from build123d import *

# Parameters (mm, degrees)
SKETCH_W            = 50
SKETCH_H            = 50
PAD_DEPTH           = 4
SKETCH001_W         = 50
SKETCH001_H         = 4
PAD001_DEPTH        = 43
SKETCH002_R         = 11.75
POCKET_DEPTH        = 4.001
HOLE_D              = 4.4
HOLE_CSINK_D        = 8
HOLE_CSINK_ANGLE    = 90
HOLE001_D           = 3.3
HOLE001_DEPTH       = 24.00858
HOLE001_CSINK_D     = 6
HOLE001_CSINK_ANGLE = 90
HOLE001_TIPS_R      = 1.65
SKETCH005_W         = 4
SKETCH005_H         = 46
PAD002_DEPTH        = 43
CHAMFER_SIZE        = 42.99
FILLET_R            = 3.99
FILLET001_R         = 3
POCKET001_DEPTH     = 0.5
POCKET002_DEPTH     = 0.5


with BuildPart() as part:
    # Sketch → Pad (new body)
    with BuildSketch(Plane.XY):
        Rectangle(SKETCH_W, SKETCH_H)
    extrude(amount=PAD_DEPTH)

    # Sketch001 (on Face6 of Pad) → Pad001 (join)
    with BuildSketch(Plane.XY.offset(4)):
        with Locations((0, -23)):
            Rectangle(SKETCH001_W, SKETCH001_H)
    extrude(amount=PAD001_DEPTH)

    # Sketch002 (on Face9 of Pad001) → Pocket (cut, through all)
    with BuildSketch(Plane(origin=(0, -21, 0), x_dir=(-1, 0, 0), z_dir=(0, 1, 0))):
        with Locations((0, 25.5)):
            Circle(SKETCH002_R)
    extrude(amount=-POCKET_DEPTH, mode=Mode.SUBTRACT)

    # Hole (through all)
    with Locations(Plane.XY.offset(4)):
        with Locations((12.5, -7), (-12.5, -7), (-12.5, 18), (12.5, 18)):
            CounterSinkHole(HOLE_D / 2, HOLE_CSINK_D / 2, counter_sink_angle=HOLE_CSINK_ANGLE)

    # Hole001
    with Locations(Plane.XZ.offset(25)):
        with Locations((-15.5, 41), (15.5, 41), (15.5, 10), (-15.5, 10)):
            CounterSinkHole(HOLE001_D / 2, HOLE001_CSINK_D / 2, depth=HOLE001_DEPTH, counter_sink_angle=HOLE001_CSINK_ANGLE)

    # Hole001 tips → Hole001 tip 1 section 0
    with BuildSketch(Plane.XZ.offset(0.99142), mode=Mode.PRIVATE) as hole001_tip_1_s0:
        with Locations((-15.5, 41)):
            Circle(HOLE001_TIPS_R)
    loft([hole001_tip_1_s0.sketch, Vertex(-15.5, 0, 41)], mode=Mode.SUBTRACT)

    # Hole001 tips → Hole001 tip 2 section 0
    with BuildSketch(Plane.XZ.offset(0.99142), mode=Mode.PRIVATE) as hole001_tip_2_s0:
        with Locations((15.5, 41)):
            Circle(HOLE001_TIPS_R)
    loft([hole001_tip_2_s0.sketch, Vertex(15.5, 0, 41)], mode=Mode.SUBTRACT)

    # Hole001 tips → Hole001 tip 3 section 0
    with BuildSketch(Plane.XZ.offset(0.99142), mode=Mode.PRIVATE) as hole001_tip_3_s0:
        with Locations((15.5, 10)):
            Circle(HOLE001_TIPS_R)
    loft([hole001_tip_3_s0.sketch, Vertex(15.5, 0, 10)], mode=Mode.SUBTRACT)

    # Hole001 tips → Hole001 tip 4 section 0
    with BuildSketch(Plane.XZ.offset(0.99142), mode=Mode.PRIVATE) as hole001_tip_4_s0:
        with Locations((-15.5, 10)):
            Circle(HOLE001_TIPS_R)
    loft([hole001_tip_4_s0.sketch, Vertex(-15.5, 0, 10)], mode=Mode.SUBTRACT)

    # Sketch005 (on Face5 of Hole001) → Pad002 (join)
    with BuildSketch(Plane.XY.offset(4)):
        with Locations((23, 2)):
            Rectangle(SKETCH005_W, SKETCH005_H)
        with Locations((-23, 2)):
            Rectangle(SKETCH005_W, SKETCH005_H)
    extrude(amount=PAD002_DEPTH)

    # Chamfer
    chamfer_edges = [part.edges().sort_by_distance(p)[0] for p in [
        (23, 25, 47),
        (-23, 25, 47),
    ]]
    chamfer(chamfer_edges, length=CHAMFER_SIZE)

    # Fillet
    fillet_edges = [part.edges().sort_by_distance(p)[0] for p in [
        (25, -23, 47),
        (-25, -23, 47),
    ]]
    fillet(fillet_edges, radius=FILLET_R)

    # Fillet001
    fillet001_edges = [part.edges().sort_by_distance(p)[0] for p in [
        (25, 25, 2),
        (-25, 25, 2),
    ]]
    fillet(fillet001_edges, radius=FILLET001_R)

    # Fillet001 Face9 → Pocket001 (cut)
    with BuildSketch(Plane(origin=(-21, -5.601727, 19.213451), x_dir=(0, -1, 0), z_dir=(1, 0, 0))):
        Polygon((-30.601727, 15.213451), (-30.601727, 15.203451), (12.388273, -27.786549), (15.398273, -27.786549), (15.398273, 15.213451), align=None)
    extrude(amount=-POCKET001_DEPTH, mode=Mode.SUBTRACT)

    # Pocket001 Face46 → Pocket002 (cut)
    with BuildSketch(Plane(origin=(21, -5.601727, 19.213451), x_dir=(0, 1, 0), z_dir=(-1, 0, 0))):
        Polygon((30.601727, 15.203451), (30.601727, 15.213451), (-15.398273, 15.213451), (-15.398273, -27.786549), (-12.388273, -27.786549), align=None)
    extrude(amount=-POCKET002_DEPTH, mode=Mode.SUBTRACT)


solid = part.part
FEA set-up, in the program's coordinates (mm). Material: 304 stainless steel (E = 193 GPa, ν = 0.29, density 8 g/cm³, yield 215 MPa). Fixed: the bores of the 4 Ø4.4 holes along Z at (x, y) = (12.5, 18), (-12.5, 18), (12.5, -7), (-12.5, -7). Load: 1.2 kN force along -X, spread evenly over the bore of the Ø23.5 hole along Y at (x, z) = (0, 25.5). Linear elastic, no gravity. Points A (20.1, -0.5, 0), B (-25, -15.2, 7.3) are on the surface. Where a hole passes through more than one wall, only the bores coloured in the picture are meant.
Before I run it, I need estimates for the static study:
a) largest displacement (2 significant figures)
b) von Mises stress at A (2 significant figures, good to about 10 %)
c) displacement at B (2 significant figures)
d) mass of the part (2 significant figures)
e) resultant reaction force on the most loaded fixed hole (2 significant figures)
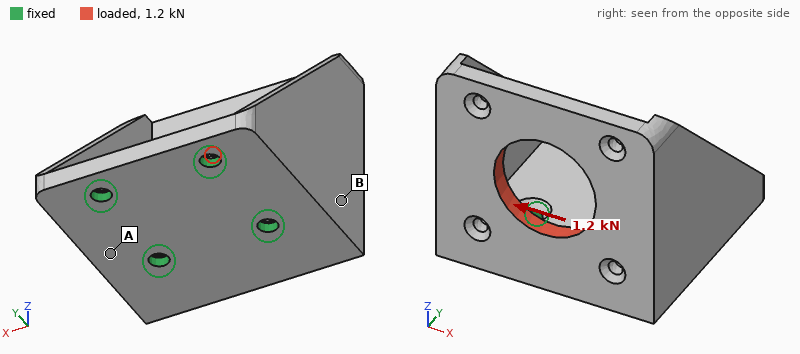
68 µm
41 MPa
24 µm
190 g
1.4 kN
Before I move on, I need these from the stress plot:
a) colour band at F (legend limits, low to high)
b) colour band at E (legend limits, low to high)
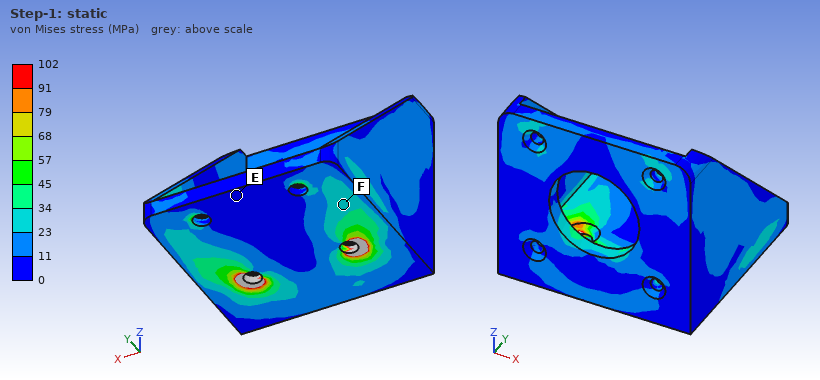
23 to 34 MPa
0 to 11 MPa
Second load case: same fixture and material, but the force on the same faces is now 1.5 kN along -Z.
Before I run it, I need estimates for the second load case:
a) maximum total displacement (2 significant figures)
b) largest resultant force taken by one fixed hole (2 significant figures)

39 µm
1.2 kN
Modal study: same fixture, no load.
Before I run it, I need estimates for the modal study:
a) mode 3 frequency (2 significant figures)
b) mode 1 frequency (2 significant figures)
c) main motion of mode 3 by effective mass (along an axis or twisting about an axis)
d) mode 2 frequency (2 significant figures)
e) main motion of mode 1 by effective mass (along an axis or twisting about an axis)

5100 Hz
2400 Hz
along Z
3100 Hz
along X
